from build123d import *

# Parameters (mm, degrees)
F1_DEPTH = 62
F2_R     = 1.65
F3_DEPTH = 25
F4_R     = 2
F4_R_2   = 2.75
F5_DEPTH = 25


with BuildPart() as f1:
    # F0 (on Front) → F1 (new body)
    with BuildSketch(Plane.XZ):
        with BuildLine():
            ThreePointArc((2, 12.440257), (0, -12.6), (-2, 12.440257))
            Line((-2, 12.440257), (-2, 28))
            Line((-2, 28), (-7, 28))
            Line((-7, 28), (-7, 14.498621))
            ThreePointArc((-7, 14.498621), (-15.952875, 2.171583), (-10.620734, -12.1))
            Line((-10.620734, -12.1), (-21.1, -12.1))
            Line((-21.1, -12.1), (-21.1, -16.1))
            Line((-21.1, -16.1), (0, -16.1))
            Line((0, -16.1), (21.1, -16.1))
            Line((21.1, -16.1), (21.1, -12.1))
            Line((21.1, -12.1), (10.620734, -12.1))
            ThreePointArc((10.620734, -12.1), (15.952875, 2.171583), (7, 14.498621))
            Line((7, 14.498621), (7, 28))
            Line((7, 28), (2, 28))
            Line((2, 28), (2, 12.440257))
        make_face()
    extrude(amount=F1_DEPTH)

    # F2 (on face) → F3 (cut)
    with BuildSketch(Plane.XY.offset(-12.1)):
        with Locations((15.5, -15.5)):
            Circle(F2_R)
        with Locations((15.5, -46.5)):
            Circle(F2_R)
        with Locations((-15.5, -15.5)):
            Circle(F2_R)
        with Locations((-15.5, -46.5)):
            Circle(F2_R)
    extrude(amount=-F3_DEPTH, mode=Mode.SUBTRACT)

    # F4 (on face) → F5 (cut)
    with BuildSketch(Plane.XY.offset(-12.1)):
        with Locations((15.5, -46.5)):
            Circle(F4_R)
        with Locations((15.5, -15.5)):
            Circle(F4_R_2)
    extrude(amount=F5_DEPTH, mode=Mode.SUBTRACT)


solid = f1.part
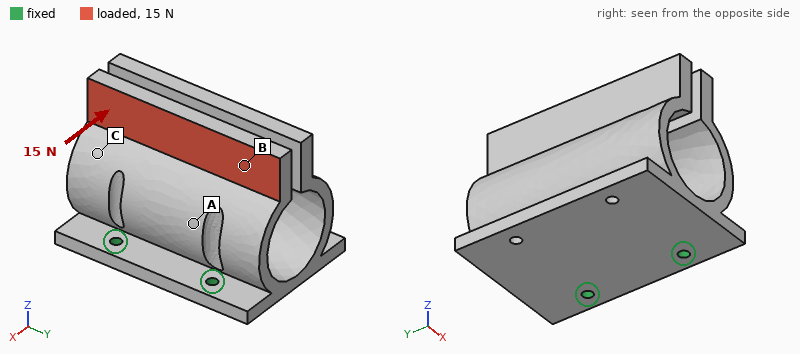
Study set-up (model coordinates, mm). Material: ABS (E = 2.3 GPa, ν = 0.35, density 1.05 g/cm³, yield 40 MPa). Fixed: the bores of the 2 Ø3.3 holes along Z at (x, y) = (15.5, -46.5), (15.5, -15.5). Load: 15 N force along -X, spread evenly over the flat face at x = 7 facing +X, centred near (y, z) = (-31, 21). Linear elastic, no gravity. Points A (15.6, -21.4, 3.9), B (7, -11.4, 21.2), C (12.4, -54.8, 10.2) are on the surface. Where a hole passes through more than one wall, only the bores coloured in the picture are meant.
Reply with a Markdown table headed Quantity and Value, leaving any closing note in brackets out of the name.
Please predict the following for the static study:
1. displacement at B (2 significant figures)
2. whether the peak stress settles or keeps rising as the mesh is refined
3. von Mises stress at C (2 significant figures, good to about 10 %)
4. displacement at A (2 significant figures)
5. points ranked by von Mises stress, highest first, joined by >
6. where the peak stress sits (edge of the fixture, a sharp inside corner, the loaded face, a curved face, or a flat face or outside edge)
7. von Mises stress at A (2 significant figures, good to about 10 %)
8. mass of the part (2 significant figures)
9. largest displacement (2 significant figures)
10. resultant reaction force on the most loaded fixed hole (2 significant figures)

| Quantity | Value |
|---|---|
| displacement at B | 0.66 mm |
| whether the peak stress settles or keeps rising as the mesh is refined | keeps rising |
| von Mises stress at C | 1.3 MPa |
| displacement at A | 0.25 mm |
| points ranked by von Mises stress, highest first, joined by > | A > C > B |
| where the peak stress sits | edge of the fixture |
| von Mises stress at A | 2.2 MPa |
| mass of the part | 35 g |
| largest displacement | 0.85 mm |
| resultant reaction force on the most loaded fixed hole | 7.6 N |
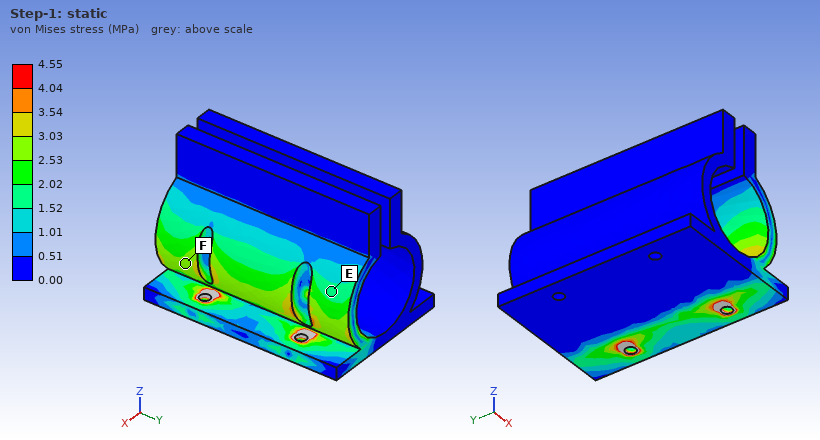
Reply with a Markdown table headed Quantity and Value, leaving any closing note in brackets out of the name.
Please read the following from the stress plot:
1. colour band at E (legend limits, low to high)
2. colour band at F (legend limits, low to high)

| Quantity | Value |
|---|---|
| colour band at E | 1.52 to 2.02 MPa |
| colour band at F | 2.53 to 3.03 MPa |
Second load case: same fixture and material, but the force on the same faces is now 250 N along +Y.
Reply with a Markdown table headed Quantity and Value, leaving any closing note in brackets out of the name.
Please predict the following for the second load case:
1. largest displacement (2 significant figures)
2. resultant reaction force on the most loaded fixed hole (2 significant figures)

| Quantity | Value |
|---|---|
| largest displacement | 0.74 mm |
| resultant reaction force on the most loaded fixed hole | 290 N |
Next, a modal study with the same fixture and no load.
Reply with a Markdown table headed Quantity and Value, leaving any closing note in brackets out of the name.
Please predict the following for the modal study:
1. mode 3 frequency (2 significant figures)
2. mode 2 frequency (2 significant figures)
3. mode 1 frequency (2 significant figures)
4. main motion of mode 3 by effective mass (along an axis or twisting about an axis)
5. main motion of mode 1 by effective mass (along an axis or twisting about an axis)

| Quantity | Value |
|---|---|
| mode 3 frequency | 430 Hz |
| mode 2 frequency | 340 Hz |
| mode 1 frequency | 220 Hz |
| main motion of mode 3 by effective mass | along Y |
| main motion of mode 1 by effective mass | along X |
